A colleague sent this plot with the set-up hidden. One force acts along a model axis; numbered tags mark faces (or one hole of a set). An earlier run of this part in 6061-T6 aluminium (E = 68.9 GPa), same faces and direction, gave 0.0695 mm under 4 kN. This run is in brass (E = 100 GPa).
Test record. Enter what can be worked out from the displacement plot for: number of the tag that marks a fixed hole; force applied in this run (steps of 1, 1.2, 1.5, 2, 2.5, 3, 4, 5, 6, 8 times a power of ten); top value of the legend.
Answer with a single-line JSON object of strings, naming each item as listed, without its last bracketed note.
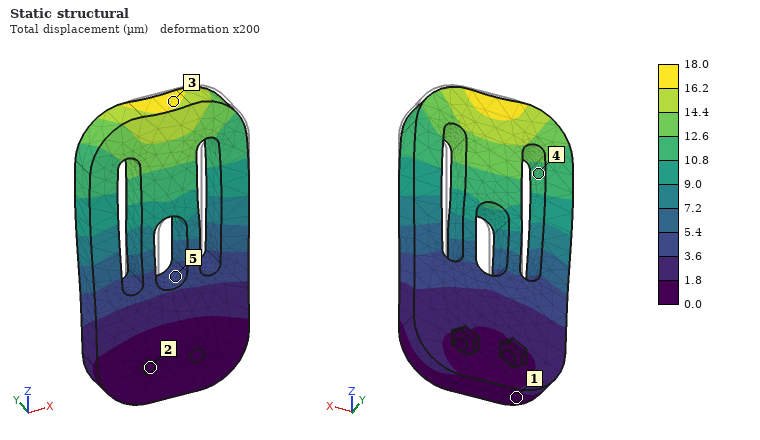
{"number of the tag that marks a fixed hole": "2", "force applied in this run": "1.5 kN", "top value of the legend": "18.0 µm"}
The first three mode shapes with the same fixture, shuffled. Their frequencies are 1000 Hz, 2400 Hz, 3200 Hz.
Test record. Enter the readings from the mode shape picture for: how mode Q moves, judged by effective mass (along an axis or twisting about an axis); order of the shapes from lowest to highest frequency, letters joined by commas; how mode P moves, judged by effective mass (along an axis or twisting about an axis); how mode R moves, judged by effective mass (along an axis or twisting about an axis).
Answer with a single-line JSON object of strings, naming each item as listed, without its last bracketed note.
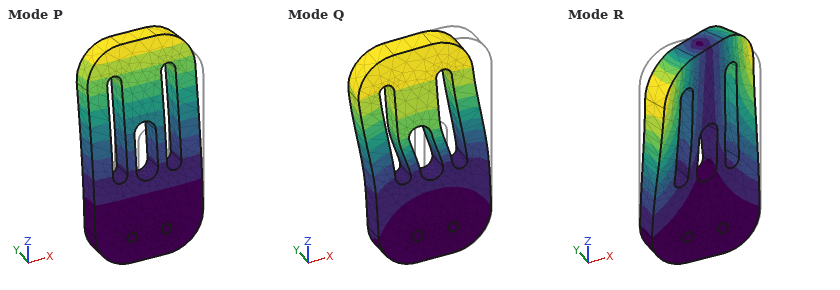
{"how mode Q moves, judged by effective mass": "along X", "order of the shapes from lowest to highest frequency, letters joined by commas": "P, Q, R", "how mode P moves, judged by effective mass": "along Y", "how mode R moves, judged by effective mass": "twisting about Z"}
